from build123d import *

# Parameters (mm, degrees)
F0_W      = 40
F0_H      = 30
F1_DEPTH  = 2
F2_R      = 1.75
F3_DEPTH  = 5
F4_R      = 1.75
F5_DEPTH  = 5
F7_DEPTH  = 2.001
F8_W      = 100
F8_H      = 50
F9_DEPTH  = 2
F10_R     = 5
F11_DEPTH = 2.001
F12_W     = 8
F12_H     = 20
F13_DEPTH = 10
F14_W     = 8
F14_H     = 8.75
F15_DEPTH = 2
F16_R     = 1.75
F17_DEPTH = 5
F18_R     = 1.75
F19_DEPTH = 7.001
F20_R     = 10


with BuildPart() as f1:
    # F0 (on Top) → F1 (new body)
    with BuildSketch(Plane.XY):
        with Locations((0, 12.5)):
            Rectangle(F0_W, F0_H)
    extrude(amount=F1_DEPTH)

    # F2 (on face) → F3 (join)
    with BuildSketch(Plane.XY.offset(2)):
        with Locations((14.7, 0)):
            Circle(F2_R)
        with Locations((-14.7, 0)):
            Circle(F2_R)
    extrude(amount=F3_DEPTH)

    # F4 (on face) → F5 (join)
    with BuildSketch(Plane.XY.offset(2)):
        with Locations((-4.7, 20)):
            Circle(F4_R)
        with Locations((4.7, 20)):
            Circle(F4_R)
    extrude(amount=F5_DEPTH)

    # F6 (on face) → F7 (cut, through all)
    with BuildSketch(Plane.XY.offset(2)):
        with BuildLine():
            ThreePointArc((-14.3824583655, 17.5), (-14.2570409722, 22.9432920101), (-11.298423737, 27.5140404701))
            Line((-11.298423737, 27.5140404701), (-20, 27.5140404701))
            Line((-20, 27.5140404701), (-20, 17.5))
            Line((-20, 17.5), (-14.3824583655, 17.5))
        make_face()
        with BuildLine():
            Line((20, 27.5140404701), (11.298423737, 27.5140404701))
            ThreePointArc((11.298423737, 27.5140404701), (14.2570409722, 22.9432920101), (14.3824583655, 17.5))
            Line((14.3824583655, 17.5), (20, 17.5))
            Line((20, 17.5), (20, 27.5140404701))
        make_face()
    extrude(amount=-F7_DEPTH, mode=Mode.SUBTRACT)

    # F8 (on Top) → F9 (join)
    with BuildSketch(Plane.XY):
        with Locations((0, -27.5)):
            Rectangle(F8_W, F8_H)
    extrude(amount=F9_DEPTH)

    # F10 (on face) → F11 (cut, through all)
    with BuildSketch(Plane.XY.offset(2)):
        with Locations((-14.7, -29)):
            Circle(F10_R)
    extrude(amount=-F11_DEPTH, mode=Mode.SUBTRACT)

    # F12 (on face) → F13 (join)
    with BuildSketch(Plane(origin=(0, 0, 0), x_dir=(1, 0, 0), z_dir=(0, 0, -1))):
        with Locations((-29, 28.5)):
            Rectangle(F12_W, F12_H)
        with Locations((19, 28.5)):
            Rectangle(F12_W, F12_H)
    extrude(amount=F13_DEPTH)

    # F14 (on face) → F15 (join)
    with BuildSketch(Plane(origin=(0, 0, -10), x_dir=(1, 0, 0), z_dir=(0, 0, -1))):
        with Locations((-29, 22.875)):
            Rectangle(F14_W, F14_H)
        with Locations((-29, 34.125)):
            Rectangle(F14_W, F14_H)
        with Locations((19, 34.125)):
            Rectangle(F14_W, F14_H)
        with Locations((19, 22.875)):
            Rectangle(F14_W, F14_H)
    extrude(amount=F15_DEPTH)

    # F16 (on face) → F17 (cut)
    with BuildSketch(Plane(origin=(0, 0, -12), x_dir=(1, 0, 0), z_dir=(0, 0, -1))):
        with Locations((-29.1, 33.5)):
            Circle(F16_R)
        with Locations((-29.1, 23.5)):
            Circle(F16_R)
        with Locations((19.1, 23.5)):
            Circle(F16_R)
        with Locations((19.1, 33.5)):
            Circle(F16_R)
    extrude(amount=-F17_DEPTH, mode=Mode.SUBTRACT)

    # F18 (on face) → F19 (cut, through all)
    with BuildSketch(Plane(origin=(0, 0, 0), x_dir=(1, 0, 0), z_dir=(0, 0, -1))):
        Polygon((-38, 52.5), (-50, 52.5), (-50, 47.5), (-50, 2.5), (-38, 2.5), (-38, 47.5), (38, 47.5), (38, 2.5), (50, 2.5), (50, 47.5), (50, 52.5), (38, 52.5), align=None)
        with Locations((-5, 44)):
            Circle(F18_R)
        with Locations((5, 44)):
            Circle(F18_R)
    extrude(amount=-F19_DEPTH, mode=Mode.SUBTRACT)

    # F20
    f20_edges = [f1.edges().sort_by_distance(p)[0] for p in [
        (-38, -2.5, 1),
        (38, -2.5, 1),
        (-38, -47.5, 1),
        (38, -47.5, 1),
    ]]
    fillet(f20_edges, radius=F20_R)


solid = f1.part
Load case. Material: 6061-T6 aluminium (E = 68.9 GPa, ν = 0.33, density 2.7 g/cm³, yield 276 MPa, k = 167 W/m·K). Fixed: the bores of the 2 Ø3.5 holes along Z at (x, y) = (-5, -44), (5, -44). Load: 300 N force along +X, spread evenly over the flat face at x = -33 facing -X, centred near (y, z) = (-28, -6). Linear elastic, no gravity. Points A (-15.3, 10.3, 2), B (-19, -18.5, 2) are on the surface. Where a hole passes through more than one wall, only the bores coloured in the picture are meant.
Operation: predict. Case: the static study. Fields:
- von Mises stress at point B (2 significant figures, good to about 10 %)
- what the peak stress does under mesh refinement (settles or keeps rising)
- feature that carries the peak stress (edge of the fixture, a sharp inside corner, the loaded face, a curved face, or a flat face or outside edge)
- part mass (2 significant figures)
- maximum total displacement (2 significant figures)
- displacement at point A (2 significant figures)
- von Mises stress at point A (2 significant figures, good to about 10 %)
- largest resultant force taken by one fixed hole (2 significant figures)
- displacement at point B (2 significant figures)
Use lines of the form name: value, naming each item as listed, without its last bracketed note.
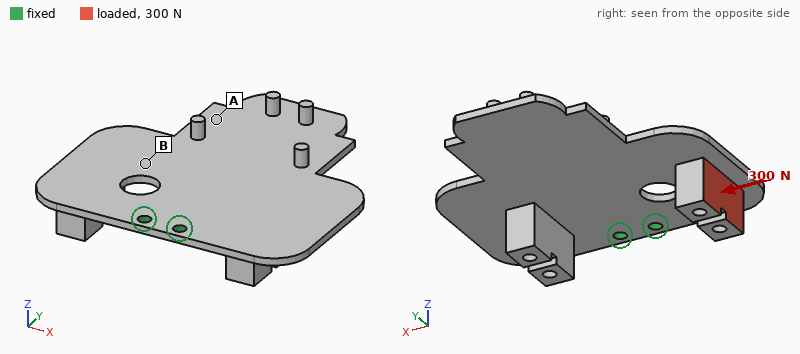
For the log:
von Mises stress at point B: 63 MPa
what the peak stress does under mesh refinement: keeps rising
feature that carries the peak stress: edge of the fixture
part mass: 33 g
maximum total displacement: 0.79 mm
displacement at point A: 0.20 mm
von Mises stress at point A: 13 MPa
largest resultant force taken by one fixed hole: 400 N
displacement at point B: 0.25 mm
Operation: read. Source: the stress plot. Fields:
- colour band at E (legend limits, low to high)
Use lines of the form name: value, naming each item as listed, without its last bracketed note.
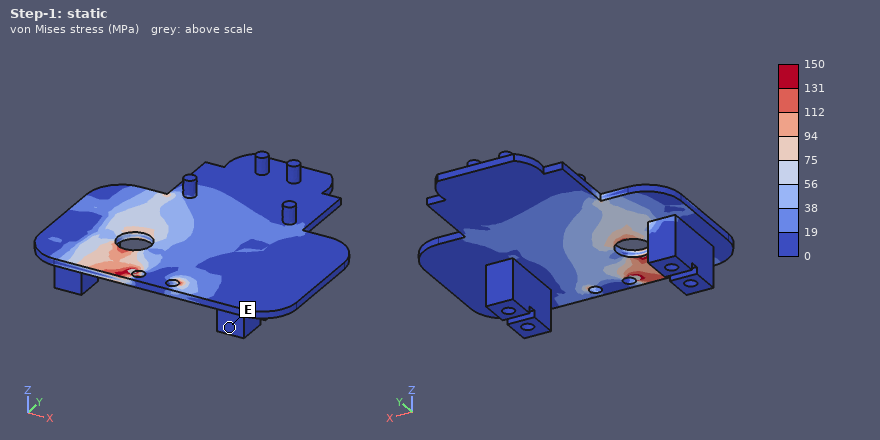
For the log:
colour band at E: 0 to 19 MPa
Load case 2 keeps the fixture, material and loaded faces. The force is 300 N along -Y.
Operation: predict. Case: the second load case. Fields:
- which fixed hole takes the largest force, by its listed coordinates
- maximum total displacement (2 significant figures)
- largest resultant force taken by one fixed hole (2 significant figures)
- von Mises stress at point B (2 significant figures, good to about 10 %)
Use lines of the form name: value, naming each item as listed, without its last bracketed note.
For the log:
which fixed hole takes the largest force, by its listed coordinates: (-5, -44)
maximum total displacement: 0.92 mm
largest resultant force taken by one fixed hole: 870 N
von Mises stress at point B: 23 MPa
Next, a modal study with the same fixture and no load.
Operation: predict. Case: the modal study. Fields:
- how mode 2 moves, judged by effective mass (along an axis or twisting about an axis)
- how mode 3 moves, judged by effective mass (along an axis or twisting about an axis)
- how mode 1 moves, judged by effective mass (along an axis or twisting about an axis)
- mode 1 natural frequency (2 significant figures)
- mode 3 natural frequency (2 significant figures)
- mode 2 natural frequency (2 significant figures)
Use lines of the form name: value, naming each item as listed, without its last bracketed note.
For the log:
how mode 2 moves, judged by effective mass: twisting about Y
how mode 3 moves, judged by effective mass: along Z
how mode 1 moves, judged by effective mass: along Z
mode 1 natural frequency: 380 Hz
mode 3 natural frequency: 1100 Hz
mode 2 natural frequency: 620 Hz
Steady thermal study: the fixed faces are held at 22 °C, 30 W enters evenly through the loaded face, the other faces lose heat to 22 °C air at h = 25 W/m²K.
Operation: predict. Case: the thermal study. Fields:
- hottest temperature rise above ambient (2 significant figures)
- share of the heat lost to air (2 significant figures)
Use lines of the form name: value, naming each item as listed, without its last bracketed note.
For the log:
hottest temperature rise above ambient: 79 K
share of the heat lost to air: 28 %
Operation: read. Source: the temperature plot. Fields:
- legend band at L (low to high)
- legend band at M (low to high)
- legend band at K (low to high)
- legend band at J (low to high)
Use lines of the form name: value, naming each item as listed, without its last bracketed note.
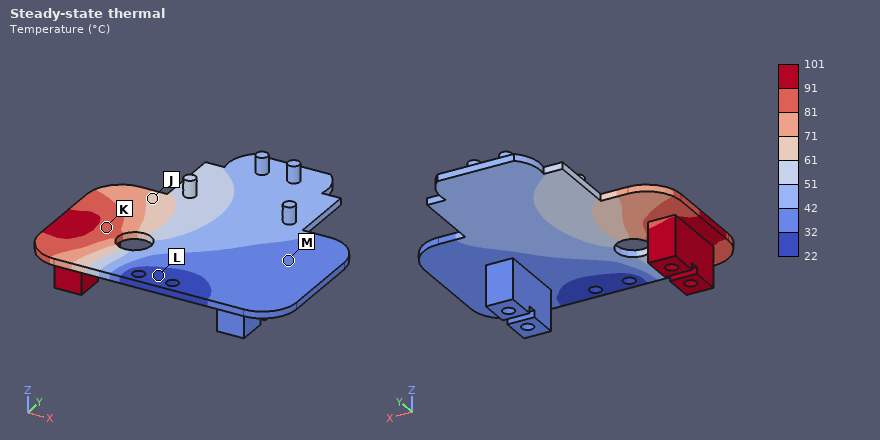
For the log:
legend band at L: 22 to 32 °C
legend band at M: 32 to 42 °C
legend band at K: 81 to 91 °C
legend band at J: 61 to 71 °C
